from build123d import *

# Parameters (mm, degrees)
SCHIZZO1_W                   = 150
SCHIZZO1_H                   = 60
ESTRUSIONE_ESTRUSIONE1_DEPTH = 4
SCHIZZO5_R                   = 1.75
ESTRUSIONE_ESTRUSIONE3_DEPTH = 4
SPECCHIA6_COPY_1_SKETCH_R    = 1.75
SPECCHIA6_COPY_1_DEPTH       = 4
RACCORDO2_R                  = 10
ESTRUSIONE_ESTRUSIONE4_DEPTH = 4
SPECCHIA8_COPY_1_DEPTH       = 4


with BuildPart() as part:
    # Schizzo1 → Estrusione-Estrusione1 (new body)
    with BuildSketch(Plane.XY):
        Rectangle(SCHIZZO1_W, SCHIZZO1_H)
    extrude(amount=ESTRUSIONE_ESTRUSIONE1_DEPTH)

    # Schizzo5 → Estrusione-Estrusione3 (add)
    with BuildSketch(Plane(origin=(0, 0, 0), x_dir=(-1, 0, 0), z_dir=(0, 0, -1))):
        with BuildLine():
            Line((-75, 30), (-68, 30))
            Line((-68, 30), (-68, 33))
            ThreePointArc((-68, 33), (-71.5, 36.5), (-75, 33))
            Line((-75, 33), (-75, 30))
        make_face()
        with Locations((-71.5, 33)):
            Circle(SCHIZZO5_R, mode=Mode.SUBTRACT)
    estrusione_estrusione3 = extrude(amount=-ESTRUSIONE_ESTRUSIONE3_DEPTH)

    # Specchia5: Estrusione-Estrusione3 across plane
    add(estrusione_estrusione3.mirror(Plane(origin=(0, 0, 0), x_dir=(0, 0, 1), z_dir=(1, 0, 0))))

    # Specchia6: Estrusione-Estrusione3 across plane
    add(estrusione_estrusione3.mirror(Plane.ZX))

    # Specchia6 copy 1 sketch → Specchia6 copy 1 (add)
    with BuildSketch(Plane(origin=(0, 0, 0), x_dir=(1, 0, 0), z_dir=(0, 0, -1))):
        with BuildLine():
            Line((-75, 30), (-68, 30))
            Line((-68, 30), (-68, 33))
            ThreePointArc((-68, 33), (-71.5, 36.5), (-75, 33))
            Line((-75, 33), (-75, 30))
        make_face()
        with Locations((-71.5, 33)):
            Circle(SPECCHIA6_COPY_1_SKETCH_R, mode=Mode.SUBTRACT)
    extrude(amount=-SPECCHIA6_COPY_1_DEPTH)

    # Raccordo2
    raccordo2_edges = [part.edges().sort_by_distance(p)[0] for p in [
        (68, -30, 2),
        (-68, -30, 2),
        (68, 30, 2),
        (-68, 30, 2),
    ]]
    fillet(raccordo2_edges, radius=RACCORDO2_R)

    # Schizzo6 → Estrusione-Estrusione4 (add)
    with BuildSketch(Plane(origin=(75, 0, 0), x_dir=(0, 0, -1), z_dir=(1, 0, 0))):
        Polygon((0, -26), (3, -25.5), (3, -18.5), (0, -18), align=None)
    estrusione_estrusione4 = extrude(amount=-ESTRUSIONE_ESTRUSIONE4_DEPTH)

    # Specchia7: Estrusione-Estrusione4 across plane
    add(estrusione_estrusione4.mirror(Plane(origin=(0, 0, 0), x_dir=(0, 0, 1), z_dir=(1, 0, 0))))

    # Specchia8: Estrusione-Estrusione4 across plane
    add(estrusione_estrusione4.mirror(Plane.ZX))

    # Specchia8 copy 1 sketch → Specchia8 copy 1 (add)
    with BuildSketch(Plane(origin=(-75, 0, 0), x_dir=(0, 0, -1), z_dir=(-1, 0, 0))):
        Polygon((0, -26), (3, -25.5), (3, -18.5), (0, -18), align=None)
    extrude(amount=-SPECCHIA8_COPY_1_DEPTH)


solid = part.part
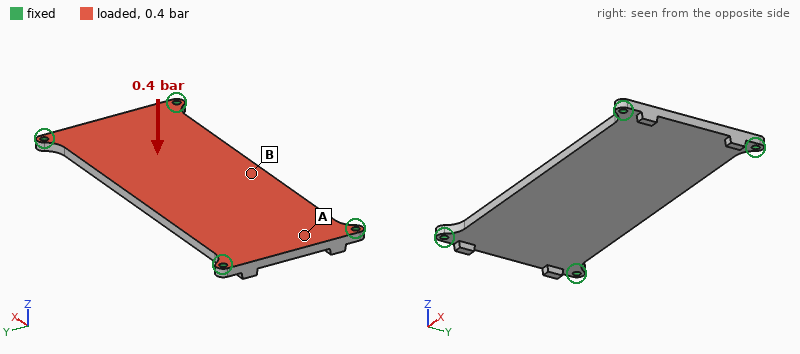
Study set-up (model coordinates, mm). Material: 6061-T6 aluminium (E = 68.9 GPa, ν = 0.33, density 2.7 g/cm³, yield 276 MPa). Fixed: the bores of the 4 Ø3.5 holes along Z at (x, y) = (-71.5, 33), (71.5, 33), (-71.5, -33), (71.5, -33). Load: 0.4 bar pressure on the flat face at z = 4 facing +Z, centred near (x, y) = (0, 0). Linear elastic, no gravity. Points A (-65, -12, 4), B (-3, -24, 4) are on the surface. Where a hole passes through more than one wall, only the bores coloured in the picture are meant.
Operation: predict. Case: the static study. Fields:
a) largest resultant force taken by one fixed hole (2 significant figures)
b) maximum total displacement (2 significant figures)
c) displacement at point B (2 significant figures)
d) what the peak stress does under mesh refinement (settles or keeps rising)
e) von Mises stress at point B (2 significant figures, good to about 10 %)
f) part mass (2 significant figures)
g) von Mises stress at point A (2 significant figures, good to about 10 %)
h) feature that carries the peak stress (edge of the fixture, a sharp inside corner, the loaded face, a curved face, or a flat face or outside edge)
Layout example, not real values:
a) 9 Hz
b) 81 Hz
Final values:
a) 92 N
b) 0.21 mm
c) 0.21 mm
d) keeps rising
e) 18 MPa
f) 100 g
g) 8.7 MPa
h) edge of the fixture
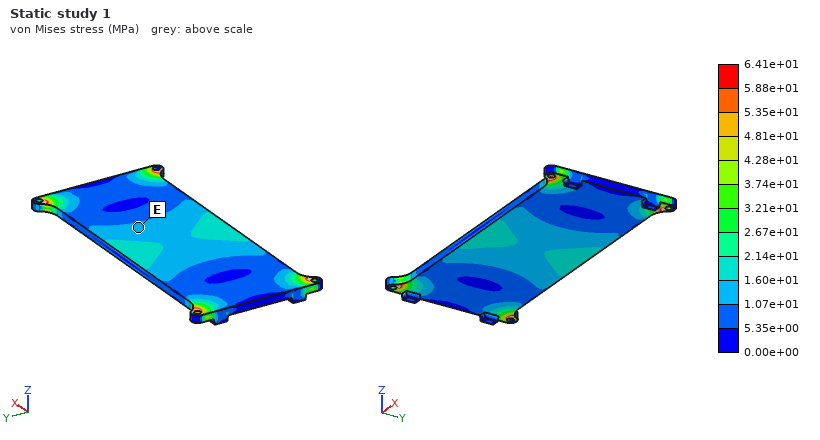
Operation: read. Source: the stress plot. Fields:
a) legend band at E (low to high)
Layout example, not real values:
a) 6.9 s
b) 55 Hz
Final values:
a) 1.07e+01 to 1.60e+01 MPa
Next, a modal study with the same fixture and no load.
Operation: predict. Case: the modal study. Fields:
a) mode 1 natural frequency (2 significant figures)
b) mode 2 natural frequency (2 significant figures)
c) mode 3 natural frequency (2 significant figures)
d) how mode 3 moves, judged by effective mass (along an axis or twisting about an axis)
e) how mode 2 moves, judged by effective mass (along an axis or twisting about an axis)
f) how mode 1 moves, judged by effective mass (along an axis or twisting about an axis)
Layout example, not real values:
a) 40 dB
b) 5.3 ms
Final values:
a) 770 Hz
b) 1800 Hz
c) 2200 Hz
d) twisting about Y
e) twisting about X
f) along Z
